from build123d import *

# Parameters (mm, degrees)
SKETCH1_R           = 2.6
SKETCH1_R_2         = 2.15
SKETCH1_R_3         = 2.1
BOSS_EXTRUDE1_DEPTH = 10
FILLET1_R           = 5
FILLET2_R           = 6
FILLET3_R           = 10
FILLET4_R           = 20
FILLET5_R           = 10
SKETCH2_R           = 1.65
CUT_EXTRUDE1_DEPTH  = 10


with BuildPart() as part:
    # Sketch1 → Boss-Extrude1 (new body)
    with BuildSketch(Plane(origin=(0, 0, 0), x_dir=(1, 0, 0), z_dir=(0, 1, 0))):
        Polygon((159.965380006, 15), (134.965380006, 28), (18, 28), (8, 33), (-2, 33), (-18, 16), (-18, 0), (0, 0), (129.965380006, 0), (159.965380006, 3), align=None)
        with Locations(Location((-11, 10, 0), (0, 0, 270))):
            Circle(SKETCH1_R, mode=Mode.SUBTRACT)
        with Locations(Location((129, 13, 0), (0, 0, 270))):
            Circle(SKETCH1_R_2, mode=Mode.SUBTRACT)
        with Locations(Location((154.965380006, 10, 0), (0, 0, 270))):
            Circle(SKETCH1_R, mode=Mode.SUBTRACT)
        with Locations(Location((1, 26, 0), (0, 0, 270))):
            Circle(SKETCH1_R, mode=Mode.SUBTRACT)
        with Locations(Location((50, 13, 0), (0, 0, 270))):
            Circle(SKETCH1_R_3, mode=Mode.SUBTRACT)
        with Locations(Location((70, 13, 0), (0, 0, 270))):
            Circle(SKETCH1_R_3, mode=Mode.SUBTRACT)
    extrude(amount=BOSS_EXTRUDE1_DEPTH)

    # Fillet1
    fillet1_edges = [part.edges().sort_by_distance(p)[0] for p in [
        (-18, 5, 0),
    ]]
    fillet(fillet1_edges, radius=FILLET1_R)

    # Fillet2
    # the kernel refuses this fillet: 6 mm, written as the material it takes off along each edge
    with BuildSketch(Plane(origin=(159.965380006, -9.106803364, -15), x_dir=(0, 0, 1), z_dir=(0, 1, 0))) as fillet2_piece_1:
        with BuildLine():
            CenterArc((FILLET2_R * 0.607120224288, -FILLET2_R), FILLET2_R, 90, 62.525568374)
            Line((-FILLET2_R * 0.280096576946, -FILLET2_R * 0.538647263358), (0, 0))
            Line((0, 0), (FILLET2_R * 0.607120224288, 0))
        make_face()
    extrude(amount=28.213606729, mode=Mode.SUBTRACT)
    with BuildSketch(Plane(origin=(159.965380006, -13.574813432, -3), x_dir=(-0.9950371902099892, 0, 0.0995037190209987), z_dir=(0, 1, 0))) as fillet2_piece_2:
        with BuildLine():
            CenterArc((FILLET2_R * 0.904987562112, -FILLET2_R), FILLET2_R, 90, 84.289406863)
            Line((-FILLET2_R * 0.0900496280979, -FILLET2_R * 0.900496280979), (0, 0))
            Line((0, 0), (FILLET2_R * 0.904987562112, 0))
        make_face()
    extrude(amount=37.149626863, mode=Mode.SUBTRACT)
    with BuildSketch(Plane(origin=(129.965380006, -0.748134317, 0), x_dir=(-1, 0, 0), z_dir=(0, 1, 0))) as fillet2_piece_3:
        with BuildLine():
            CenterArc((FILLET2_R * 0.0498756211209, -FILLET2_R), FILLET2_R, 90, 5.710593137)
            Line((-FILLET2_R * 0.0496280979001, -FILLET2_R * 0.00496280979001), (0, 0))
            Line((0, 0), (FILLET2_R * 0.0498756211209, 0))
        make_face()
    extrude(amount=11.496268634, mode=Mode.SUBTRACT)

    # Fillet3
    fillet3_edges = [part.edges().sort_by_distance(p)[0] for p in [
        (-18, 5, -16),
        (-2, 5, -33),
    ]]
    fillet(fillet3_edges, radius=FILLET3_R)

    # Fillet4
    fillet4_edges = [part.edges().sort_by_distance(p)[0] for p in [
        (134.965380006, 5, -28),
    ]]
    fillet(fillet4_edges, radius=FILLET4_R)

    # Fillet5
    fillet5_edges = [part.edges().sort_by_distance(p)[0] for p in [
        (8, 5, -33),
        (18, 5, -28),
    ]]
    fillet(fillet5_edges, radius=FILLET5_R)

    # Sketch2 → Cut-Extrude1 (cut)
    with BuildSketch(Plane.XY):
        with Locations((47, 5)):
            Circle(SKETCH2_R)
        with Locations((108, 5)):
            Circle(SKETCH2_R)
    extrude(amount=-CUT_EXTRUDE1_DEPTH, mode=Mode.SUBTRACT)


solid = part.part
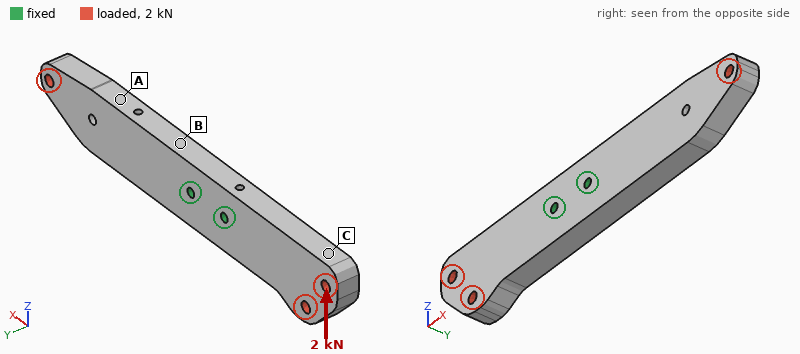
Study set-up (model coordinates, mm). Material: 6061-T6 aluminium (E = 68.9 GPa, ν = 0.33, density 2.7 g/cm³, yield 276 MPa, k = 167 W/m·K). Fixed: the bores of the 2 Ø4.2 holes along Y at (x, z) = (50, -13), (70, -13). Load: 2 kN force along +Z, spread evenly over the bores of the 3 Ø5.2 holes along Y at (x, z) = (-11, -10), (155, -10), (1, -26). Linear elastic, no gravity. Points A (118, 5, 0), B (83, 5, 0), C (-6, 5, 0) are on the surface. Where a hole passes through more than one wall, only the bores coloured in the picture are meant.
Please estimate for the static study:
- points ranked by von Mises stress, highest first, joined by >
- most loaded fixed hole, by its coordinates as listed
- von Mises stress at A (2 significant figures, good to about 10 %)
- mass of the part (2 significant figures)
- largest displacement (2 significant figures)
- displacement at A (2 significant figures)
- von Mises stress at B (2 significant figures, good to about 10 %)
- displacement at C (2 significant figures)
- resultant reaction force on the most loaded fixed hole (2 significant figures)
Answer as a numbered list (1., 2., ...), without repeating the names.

1. B > A > C
2. (50, -13)
3. 18 MPa
4. 130 g
5. 0.16 mm
6. 0.070 mm
7. 36 MPa
8. 0.11 mm
9. 2.1 kN
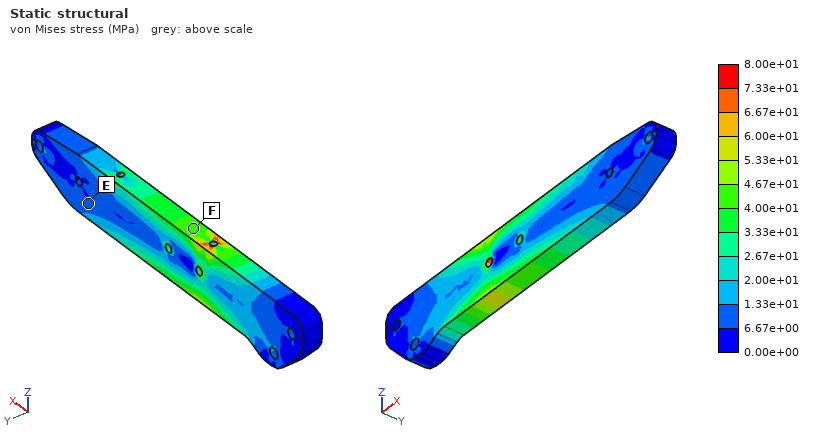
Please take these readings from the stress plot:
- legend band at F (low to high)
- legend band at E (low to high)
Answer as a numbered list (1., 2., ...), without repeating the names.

1. 4.00e+01 to 4.67e+01 MPa
2. 6.67e+00 to 1.33e+01 MPa
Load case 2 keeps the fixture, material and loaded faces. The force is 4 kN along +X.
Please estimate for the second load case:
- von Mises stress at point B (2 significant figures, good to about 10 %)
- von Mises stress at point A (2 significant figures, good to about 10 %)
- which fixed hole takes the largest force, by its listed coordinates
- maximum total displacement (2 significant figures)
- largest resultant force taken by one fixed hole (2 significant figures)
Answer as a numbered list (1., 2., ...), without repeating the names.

1. 7.1 MPa
2. 8.8 MPa
3. (50, -13)
4. 27 µm
5. 2.3 kN
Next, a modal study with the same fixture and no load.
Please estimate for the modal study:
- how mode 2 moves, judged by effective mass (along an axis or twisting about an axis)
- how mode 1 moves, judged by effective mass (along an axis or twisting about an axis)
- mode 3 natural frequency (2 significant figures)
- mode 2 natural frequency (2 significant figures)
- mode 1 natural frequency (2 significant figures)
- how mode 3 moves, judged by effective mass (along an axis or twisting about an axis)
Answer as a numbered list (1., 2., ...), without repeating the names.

1. along Y
2. along Y
3. 2400 Hz
4. 1800 Hz
5. 1100 Hz
6. along Z
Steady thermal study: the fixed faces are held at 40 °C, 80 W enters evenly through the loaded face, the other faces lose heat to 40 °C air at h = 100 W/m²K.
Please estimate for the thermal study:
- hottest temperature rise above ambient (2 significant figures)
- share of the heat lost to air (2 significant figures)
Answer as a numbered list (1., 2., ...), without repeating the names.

1. 53 K
2. 35 %
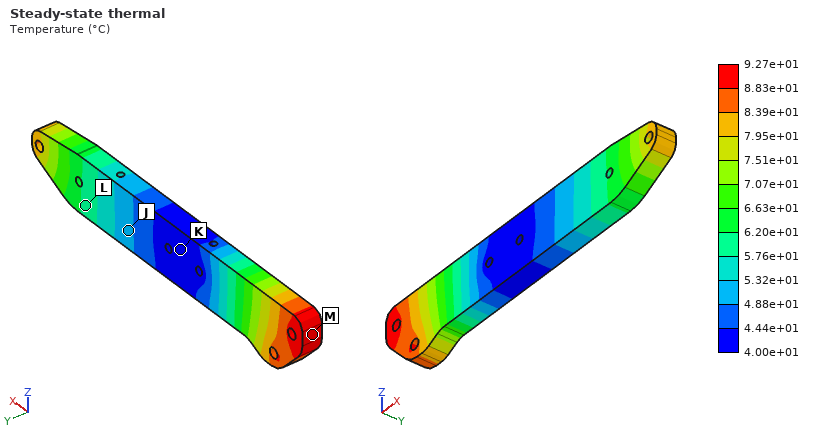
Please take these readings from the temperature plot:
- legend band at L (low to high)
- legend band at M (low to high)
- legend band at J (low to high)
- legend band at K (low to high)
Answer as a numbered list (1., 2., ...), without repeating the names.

1. 5.76e+01 to 6.20e+01 °C
2. 8.83e+01 to 9.27e+01 °C
3. 4.88e+01 to 5.32e+01 °C
4. 4.00e+01 to 4.44e+01 °C
